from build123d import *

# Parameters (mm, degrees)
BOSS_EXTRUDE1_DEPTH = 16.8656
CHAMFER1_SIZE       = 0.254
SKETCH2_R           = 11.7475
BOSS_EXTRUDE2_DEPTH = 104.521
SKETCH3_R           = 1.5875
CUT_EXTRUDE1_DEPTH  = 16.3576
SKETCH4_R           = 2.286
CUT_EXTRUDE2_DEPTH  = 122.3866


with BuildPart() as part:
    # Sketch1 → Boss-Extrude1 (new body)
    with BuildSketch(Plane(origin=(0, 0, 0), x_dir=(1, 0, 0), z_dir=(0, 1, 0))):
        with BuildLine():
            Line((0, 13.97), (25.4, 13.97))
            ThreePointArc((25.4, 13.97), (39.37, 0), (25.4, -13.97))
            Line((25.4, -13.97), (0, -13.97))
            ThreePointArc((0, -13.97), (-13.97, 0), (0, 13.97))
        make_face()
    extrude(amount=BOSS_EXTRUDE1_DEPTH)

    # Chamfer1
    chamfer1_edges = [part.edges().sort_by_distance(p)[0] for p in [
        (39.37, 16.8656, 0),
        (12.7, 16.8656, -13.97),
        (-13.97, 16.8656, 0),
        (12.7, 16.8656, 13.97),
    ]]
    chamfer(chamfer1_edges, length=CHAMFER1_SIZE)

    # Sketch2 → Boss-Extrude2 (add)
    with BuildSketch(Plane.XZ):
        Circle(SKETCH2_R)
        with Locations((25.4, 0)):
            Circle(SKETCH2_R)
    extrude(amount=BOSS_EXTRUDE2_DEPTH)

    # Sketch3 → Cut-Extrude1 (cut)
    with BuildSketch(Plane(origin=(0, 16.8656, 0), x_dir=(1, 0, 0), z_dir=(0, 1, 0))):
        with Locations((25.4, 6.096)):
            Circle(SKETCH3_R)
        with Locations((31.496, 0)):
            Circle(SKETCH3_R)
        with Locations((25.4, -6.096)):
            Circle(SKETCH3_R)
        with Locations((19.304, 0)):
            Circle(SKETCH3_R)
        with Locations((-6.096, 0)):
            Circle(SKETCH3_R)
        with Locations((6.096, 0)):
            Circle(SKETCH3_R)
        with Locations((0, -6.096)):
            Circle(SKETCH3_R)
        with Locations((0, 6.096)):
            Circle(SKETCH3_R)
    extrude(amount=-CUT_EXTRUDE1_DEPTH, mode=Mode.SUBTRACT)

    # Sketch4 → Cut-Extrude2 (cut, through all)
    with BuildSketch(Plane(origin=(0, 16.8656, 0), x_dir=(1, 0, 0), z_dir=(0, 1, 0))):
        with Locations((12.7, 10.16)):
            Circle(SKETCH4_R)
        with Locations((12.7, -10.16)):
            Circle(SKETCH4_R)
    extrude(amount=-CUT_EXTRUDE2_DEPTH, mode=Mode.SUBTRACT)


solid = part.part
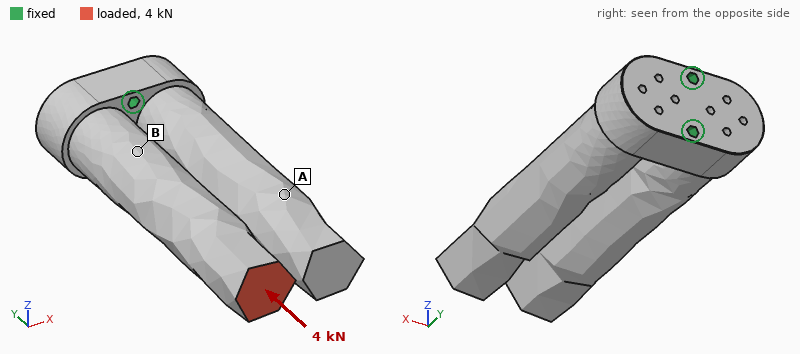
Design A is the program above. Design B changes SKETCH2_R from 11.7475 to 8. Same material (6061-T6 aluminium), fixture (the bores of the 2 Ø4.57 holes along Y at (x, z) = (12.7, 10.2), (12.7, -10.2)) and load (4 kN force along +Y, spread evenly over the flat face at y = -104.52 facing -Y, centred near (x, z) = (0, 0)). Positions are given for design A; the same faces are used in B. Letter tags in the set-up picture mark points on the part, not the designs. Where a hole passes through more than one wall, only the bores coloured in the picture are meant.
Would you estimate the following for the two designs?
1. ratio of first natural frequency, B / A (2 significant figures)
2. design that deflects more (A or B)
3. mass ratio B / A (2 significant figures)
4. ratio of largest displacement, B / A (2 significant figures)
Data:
0.83
B
0.56
1.1
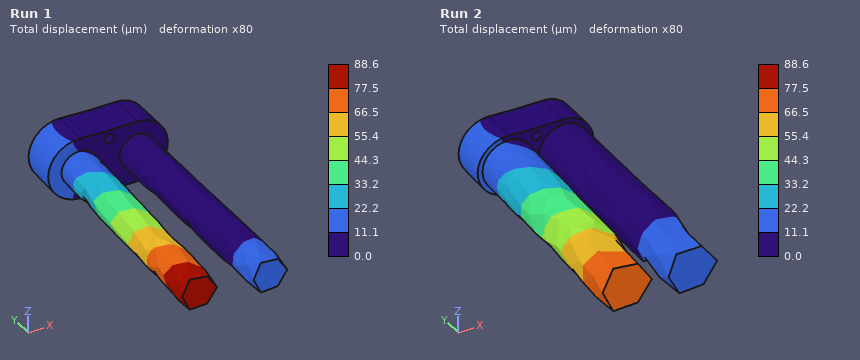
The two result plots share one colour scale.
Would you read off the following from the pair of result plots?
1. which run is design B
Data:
Run 1
